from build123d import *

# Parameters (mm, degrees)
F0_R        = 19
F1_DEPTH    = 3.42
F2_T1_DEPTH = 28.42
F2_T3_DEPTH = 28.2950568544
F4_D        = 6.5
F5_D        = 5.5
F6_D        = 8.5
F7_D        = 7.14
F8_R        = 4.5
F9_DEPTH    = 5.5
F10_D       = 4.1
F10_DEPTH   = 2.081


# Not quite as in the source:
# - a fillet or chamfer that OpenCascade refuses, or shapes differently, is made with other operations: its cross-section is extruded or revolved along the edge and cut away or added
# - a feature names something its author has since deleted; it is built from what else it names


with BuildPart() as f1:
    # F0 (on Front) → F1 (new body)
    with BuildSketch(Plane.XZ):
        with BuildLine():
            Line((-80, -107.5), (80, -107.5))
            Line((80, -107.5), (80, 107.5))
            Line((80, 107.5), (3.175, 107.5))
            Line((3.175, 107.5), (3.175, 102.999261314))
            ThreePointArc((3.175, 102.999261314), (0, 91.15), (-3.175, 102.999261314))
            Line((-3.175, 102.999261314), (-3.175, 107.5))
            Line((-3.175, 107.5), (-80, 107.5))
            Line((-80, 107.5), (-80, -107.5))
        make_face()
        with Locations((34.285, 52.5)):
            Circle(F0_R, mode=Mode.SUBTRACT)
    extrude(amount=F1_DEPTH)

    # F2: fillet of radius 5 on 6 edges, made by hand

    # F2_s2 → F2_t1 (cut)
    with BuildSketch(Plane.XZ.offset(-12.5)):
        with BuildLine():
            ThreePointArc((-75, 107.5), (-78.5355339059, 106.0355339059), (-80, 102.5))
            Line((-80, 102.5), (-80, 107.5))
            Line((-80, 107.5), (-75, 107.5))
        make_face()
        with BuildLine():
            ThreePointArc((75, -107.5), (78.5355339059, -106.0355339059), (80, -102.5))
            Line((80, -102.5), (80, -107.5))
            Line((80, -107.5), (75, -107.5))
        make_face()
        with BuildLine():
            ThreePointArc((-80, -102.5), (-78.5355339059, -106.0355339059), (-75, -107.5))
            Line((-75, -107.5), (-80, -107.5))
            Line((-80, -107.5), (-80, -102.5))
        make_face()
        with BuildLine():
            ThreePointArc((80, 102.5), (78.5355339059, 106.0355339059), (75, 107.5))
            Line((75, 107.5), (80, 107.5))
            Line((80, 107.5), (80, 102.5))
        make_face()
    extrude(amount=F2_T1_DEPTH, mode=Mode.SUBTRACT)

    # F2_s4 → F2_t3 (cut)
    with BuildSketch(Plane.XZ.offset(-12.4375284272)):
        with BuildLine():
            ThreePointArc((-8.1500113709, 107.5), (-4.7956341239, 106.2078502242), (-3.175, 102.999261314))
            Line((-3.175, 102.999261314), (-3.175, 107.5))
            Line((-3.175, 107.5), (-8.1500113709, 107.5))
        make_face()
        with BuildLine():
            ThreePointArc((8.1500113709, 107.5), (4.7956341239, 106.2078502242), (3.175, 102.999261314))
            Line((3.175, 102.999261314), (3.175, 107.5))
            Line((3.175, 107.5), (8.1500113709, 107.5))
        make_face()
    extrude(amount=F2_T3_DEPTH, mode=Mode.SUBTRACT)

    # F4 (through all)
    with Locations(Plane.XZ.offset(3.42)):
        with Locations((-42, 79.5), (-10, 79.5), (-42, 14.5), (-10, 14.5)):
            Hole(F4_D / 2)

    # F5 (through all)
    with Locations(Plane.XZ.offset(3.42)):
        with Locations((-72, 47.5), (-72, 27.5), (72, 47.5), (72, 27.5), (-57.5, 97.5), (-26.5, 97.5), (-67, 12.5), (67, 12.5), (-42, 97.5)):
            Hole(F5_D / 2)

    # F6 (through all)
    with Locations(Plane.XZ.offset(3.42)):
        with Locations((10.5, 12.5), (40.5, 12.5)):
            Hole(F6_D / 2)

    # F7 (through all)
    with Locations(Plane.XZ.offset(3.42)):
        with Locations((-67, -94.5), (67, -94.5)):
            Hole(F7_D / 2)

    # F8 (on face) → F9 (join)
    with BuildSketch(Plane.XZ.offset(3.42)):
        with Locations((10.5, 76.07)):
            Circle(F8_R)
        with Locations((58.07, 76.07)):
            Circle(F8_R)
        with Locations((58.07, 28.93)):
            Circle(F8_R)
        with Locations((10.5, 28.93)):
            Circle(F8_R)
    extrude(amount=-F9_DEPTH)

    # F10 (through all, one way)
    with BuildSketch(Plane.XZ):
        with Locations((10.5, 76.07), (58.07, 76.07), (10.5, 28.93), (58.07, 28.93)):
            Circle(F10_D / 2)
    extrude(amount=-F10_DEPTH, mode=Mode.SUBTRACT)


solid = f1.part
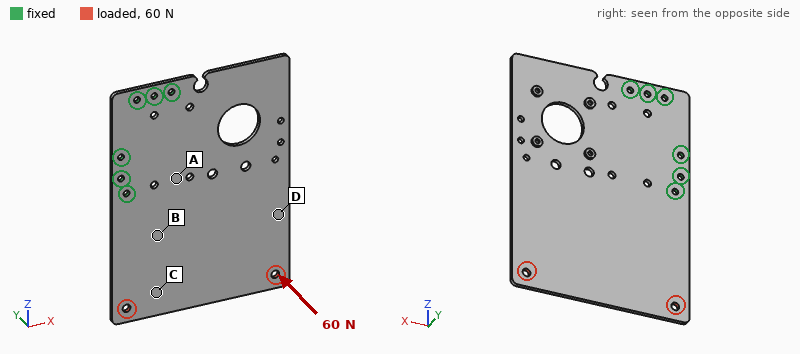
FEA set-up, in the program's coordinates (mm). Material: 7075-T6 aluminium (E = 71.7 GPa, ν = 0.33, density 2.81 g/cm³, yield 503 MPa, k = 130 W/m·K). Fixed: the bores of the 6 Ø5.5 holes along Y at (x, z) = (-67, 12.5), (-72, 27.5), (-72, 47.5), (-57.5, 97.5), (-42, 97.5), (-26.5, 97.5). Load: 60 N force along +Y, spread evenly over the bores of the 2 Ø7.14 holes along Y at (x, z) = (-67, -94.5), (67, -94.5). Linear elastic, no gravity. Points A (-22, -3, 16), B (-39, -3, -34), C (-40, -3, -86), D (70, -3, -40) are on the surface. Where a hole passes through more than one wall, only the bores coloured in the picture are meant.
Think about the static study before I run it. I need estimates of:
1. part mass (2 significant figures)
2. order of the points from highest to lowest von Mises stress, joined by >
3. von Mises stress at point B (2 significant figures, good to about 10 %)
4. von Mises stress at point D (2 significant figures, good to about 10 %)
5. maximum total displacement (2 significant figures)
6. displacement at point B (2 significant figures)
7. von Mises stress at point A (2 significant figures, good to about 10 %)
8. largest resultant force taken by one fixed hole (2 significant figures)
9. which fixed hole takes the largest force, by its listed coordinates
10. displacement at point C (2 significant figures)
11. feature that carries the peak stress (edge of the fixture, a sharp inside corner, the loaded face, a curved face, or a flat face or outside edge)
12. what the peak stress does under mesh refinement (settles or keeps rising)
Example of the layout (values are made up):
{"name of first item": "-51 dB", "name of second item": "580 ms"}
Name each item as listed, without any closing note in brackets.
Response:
{"part mass": "310 g", "order of the points from highest to lowest von Mises stress, joined by >": "A > B > D > C", "von Mises stress at point B": "13 MPa", "von Mises stress at point D": "8.7 MPa", "maximum total displacement": "2.4 mm", "displacement at point B": "0.45 mm", "von Mises stress at point A": "21 MPa", "largest resultant force taken by one fixed hole": "190 N", "which fixed hole takes the largest force, by its listed coordinates": "(-67, 12.5)", "displacement at point C": "1.1 mm", "feature that carries the peak stress": "edge of the fixture", "what the peak stress does under mesh refinement": "keeps rising"}
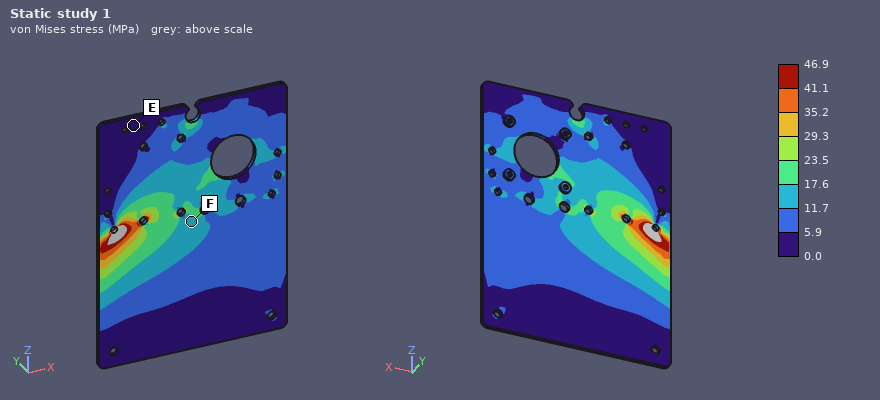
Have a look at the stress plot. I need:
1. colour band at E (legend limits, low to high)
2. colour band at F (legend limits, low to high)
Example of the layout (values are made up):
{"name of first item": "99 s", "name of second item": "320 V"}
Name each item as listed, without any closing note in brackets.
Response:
{"colour band at E": "0.0 to 5.9 MPa", "colour band at F": "11.7 to 17.6 MPa"}
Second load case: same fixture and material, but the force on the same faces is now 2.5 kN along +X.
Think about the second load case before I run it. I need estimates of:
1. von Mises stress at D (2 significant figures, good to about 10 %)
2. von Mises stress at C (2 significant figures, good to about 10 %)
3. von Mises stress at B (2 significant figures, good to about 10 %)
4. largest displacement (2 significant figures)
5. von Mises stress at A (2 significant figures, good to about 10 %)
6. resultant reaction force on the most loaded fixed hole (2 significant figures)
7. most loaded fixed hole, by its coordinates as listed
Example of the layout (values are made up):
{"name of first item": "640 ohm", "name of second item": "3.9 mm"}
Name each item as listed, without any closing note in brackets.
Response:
{"von Mises stress at D": "7.6 MPa", "von Mises stress at C": "9.5 MPa", "von Mises stress at B": "16 MPa", "largest displacement": "0.18 mm", "von Mises stress at A": "15 MPa", "resultant reaction force on the most loaded fixed hole": "4.2 kN", "most loaded fixed hole, by its coordinates as listed": "(-67, 12.5)"}
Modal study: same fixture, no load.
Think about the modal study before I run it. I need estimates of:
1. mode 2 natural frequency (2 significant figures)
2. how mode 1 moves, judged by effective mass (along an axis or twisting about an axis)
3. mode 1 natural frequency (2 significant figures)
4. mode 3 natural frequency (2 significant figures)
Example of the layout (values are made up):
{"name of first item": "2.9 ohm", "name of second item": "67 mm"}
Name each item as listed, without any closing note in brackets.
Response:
{"mode 2 natural frequency": "200 Hz", "how mode 1 moves, judged by effective mass": "along Y", "mode 1 natural frequency": "96 Hz", "mode 3 natural frequency": "350 Hz"}
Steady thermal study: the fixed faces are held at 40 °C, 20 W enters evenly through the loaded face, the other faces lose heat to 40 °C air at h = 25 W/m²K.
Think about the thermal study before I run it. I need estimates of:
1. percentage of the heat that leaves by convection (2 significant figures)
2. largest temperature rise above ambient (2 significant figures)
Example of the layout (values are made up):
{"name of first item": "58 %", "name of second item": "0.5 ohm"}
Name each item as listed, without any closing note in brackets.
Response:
{"percentage of the heat that leaves by convection": "73 %", "largest temperature rise above ambient": "33 K"}
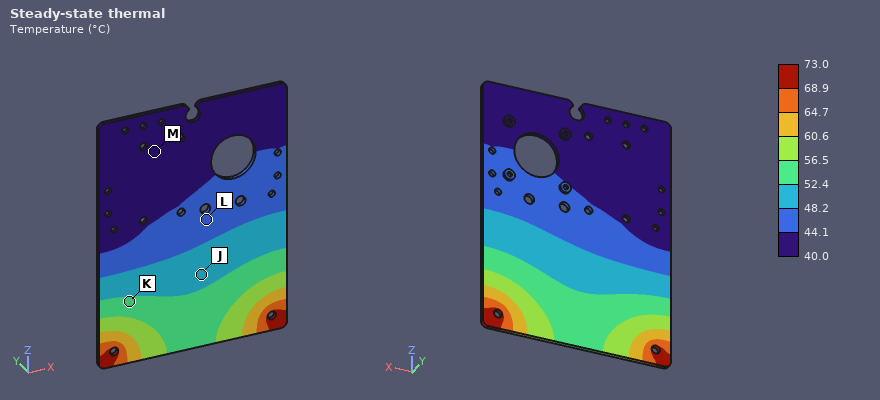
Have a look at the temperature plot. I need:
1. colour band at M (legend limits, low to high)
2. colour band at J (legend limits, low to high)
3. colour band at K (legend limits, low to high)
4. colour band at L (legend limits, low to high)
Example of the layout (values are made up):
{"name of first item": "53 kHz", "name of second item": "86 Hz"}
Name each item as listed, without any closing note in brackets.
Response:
{"colour band at M": "40.0 to 44.1 °C", "colour band at J": "48.2 to 52.4 °C", "colour band at K": "52.4 to 56.5 °C", "colour band at L": "44.1 to 48.2 °C"}
